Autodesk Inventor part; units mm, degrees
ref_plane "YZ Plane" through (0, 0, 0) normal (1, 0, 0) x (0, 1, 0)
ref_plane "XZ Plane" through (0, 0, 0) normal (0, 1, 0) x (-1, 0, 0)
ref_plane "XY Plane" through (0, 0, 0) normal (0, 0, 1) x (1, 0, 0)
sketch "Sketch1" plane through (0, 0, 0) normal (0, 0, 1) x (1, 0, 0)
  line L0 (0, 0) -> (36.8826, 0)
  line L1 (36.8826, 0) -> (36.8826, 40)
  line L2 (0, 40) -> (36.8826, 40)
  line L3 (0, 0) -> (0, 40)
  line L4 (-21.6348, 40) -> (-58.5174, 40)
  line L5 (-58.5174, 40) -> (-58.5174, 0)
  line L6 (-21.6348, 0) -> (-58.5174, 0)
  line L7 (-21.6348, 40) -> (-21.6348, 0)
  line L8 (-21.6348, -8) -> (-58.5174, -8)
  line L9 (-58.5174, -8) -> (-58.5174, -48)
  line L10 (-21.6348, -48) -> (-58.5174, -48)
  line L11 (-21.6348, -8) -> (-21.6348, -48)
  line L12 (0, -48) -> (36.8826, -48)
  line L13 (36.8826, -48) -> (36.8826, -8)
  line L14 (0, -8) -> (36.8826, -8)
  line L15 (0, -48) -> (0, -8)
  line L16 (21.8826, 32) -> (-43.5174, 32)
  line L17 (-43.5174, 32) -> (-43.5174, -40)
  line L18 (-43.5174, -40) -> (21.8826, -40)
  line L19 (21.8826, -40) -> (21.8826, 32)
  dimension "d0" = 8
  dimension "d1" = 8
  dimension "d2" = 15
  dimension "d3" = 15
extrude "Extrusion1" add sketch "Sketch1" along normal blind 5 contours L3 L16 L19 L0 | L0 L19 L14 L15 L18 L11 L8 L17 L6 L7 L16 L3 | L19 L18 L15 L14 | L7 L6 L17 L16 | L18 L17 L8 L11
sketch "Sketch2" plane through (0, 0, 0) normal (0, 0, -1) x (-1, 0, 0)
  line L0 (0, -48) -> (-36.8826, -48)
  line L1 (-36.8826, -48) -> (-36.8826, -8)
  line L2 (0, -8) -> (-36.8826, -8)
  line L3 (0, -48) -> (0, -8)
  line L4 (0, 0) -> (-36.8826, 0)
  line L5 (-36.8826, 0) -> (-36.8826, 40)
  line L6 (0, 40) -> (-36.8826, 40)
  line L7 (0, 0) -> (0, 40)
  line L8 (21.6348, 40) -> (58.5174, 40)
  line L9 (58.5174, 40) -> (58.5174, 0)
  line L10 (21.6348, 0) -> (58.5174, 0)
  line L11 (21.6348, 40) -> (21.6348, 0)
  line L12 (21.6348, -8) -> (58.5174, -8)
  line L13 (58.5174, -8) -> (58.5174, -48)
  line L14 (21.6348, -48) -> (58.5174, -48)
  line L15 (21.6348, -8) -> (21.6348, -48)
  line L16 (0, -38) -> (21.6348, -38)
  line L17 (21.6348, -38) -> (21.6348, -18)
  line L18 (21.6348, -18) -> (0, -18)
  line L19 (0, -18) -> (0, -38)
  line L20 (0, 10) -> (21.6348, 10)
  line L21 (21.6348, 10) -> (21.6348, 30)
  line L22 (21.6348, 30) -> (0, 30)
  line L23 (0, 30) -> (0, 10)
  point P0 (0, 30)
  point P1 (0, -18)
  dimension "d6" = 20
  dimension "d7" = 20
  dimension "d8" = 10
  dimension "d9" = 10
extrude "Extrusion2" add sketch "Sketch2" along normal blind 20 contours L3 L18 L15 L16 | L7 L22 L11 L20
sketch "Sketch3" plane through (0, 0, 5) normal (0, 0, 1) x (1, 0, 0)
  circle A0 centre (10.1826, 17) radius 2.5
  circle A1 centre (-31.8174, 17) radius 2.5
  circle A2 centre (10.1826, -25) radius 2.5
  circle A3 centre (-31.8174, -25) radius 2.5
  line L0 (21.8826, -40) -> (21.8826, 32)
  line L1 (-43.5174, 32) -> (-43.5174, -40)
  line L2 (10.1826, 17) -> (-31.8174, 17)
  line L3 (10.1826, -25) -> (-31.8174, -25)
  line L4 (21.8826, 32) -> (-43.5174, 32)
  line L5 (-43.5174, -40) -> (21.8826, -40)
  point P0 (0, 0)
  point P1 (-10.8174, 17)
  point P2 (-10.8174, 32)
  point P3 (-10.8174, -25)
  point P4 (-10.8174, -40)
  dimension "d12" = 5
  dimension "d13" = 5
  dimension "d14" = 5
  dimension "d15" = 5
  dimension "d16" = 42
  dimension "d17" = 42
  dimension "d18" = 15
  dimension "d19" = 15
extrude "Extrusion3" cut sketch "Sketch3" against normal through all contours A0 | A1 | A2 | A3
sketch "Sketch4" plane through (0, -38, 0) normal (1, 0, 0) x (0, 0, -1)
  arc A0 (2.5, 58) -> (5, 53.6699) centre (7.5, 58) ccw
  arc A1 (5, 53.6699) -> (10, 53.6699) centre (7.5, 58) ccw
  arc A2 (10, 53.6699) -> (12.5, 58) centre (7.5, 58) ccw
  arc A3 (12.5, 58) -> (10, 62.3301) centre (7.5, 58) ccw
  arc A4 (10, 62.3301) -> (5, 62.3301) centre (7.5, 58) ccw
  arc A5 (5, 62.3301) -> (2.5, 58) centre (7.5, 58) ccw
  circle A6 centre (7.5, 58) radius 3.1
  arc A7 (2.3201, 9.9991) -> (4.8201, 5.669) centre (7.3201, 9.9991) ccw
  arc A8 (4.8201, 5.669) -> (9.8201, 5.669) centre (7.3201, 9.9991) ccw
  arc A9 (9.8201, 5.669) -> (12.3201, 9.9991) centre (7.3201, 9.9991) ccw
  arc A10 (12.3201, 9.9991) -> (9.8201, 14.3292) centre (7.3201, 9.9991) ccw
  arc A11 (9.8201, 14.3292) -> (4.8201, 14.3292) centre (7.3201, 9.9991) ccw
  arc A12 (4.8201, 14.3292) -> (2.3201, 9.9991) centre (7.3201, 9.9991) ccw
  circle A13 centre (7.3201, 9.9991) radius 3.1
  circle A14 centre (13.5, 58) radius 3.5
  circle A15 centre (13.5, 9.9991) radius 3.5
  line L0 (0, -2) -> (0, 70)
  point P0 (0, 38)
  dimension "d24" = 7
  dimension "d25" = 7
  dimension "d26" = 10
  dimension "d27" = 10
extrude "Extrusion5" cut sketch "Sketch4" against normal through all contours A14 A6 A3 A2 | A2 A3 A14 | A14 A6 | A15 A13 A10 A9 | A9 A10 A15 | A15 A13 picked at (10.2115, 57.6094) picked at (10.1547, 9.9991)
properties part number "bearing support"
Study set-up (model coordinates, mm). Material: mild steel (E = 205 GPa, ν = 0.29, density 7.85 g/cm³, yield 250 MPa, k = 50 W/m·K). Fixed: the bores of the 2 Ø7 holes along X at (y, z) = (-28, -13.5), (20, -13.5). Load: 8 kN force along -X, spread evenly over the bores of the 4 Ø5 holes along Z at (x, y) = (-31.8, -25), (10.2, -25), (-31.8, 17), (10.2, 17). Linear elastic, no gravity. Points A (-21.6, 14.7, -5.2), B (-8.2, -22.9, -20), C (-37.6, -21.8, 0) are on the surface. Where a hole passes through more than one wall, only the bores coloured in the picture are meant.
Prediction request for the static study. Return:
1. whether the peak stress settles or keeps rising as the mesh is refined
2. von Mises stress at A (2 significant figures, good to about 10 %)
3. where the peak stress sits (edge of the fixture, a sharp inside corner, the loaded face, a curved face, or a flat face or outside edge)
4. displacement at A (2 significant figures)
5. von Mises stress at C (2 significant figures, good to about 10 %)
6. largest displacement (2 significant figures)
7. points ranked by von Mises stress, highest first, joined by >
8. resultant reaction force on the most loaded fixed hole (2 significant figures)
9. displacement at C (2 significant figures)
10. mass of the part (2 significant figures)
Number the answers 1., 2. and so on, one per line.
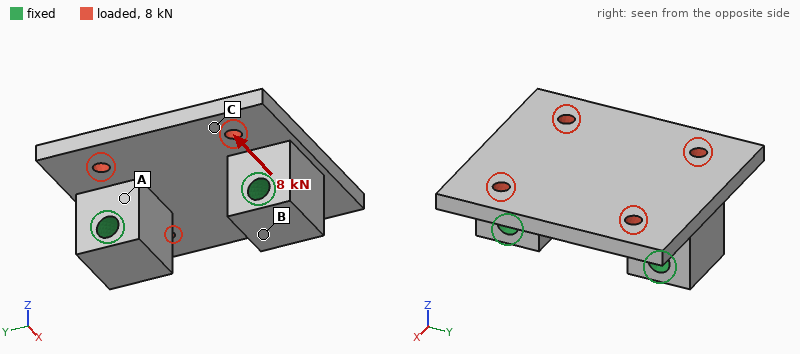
1. keeps rising
2. 23 MPa
3. edge of the fixture
4. 2.1 µm
5. 14 MPa
6. 9.1 µm
7. A > C > B
8. 4.0 kN
9. 7.2 µm
10. 300 g
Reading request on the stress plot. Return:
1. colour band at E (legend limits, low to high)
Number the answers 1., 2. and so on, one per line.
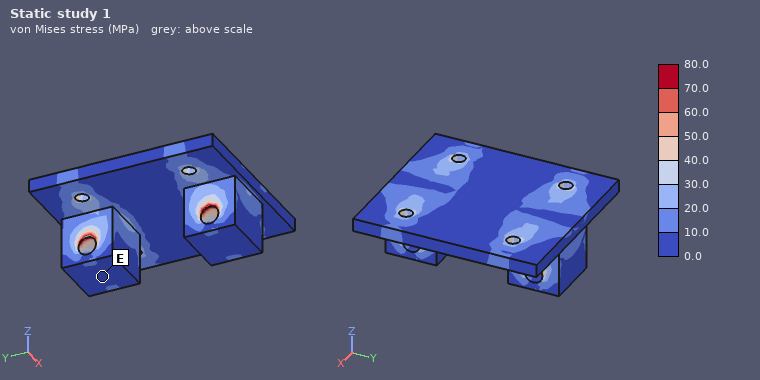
1. 0.0 to 10.0 MPa
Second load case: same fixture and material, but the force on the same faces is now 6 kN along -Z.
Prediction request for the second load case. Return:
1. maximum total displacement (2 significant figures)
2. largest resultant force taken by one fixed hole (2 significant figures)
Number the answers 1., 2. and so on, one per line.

1. 43 µm
2. 3.0 kN
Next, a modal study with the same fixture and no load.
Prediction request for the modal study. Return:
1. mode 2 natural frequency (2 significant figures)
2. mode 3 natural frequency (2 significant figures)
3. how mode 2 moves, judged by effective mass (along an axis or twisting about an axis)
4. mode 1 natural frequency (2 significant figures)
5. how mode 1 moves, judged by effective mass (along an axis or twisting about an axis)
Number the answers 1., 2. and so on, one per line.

1. 6000 Hz
2. 7900 Hz
3. along Z
4. 5600 Hz
5. twisting about Y
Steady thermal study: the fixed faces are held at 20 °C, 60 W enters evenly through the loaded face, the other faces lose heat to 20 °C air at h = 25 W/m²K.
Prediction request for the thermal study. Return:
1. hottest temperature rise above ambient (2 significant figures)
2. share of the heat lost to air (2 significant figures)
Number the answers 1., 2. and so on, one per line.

1. 51 K
2. 14 %
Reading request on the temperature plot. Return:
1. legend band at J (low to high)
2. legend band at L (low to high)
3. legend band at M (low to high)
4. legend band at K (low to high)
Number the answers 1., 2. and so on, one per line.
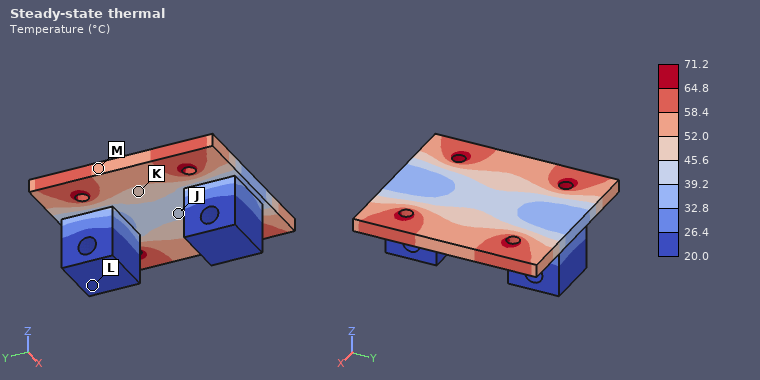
1. 39.2 to 45.6 °C
2. 20.0 to 26.4 °C
3. 52.0 to 58.4 °C
4. 45.6 to 52.0 °C
